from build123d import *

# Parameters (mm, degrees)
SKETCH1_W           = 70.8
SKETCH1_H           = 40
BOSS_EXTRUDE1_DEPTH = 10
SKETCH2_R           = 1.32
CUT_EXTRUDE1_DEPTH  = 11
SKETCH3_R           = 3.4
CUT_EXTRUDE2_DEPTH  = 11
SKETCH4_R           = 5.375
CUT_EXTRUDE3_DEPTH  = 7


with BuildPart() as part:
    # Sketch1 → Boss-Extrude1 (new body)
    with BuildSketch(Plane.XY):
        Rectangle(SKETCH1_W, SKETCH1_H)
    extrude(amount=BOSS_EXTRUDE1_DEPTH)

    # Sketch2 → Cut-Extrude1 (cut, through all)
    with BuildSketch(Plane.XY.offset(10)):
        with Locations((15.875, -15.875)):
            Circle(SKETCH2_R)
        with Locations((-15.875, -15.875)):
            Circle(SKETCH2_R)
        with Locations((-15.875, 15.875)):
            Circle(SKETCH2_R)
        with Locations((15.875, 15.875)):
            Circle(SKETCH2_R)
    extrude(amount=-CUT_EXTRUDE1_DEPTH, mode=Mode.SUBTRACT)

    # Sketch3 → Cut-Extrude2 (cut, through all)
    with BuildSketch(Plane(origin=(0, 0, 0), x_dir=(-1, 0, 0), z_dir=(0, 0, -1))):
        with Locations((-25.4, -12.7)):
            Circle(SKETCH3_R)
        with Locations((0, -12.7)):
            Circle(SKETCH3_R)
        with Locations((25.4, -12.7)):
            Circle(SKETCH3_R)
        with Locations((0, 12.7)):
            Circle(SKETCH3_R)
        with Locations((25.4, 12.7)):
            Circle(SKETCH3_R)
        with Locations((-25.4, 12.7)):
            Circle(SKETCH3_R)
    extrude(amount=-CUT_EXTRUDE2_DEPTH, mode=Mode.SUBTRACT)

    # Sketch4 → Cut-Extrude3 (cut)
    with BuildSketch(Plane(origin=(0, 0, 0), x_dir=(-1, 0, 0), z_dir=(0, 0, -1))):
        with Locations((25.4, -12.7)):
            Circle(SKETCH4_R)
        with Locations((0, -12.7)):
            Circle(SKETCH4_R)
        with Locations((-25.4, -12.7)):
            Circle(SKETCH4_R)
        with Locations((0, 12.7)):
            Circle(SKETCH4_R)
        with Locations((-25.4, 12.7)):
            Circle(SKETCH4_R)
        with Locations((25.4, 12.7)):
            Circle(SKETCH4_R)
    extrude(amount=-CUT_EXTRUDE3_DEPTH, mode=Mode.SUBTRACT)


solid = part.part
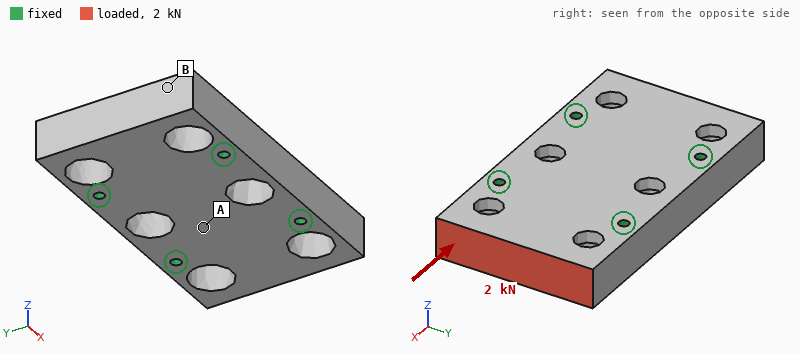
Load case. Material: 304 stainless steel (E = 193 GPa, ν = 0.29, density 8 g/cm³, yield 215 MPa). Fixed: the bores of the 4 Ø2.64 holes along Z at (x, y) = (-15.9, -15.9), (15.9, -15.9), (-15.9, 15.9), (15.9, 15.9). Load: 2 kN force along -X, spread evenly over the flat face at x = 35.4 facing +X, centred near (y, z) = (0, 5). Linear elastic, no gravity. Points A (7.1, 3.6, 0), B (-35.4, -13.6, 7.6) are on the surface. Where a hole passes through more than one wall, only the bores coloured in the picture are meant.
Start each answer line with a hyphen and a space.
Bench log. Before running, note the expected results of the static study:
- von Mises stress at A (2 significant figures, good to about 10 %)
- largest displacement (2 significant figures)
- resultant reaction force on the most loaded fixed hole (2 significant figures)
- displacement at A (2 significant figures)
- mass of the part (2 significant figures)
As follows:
- 4.9 MPa
- 2.0 µm
- 800 N
- 0.41 µm
- 190 g
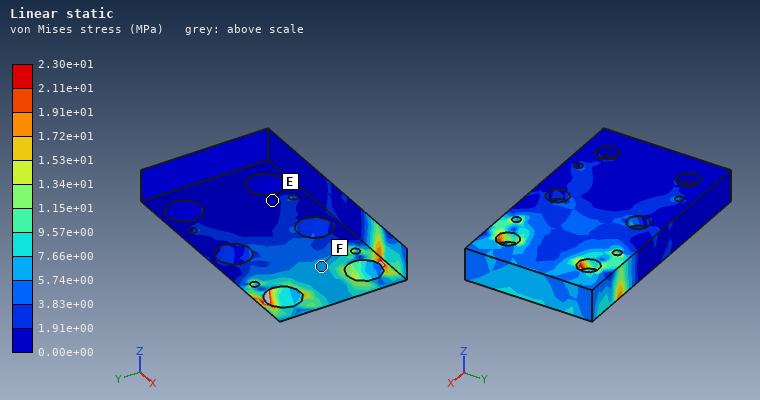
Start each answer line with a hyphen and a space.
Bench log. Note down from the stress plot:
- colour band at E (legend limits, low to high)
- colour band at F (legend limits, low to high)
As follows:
- 0.00e+00 to 1.91e+00 MPa
- 5.74e+00 to 7.66e+00 MPa
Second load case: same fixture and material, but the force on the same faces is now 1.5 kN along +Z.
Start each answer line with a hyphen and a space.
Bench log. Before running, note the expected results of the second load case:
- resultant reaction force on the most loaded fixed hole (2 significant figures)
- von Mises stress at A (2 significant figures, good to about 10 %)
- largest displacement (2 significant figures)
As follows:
- 940 N
- 20 MPa
- 17 µm
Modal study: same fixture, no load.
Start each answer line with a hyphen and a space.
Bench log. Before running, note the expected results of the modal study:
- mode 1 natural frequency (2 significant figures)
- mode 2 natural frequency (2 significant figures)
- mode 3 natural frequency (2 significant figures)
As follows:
- 12 kHz
- 12 kHz
- 20 kHz
